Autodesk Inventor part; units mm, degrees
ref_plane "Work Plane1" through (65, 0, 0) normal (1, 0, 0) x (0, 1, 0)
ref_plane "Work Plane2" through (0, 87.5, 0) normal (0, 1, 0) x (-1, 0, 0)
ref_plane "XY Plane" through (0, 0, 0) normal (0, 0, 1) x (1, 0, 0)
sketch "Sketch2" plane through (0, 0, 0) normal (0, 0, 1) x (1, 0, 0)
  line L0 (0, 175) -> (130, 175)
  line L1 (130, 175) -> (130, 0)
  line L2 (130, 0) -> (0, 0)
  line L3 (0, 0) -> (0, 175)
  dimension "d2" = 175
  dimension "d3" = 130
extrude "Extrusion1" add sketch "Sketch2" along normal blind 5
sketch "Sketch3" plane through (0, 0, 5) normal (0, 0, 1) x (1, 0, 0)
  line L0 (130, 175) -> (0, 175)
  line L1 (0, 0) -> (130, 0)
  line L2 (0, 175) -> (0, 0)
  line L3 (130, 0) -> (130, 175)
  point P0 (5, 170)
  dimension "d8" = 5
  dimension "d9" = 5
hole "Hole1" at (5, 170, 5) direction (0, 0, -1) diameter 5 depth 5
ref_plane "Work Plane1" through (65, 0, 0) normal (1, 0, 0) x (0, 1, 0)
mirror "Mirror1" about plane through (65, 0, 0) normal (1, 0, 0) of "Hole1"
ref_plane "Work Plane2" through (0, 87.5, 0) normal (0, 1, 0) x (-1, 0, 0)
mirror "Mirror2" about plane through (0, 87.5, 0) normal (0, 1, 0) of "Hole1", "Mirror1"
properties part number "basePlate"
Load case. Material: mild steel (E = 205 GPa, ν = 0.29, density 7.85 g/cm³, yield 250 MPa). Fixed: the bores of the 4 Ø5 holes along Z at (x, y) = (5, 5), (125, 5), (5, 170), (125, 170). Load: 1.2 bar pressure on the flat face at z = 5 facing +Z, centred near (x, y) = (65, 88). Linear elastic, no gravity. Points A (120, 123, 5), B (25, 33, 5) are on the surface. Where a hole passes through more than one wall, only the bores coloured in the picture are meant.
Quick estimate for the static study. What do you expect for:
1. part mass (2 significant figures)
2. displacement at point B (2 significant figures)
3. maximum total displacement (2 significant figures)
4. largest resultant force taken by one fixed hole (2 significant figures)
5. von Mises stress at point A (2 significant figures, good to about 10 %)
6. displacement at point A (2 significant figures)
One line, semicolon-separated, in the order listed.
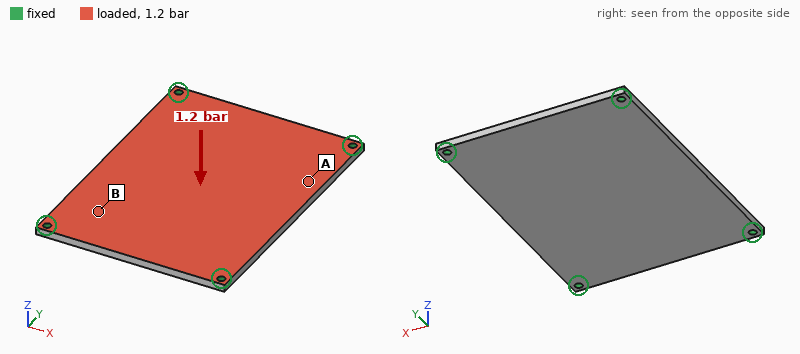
890 g; 0.10 mm; 0.23 mm; 680 N; 33 MPa; 0.14 mm
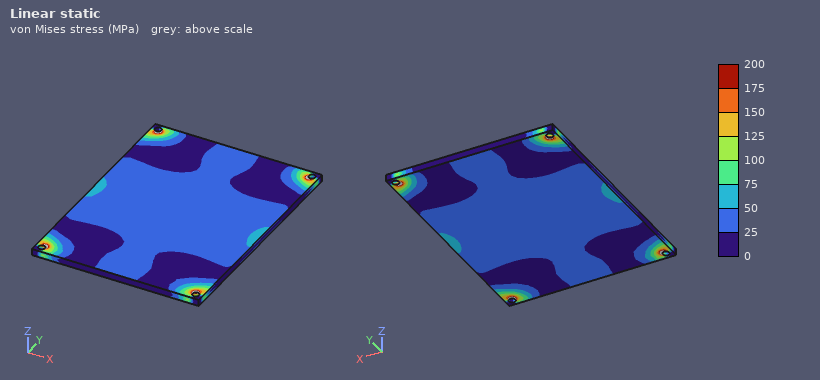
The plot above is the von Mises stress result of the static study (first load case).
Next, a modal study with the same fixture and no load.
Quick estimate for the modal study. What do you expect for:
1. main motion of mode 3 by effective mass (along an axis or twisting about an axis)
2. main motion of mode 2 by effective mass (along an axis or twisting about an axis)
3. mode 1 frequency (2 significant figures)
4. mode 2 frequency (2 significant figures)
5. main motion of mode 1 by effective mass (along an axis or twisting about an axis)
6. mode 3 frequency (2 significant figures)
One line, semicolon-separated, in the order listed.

twisting about X; twisting about Y; 680 Hz; 1200 Hz; along Z; 1600 Hz
